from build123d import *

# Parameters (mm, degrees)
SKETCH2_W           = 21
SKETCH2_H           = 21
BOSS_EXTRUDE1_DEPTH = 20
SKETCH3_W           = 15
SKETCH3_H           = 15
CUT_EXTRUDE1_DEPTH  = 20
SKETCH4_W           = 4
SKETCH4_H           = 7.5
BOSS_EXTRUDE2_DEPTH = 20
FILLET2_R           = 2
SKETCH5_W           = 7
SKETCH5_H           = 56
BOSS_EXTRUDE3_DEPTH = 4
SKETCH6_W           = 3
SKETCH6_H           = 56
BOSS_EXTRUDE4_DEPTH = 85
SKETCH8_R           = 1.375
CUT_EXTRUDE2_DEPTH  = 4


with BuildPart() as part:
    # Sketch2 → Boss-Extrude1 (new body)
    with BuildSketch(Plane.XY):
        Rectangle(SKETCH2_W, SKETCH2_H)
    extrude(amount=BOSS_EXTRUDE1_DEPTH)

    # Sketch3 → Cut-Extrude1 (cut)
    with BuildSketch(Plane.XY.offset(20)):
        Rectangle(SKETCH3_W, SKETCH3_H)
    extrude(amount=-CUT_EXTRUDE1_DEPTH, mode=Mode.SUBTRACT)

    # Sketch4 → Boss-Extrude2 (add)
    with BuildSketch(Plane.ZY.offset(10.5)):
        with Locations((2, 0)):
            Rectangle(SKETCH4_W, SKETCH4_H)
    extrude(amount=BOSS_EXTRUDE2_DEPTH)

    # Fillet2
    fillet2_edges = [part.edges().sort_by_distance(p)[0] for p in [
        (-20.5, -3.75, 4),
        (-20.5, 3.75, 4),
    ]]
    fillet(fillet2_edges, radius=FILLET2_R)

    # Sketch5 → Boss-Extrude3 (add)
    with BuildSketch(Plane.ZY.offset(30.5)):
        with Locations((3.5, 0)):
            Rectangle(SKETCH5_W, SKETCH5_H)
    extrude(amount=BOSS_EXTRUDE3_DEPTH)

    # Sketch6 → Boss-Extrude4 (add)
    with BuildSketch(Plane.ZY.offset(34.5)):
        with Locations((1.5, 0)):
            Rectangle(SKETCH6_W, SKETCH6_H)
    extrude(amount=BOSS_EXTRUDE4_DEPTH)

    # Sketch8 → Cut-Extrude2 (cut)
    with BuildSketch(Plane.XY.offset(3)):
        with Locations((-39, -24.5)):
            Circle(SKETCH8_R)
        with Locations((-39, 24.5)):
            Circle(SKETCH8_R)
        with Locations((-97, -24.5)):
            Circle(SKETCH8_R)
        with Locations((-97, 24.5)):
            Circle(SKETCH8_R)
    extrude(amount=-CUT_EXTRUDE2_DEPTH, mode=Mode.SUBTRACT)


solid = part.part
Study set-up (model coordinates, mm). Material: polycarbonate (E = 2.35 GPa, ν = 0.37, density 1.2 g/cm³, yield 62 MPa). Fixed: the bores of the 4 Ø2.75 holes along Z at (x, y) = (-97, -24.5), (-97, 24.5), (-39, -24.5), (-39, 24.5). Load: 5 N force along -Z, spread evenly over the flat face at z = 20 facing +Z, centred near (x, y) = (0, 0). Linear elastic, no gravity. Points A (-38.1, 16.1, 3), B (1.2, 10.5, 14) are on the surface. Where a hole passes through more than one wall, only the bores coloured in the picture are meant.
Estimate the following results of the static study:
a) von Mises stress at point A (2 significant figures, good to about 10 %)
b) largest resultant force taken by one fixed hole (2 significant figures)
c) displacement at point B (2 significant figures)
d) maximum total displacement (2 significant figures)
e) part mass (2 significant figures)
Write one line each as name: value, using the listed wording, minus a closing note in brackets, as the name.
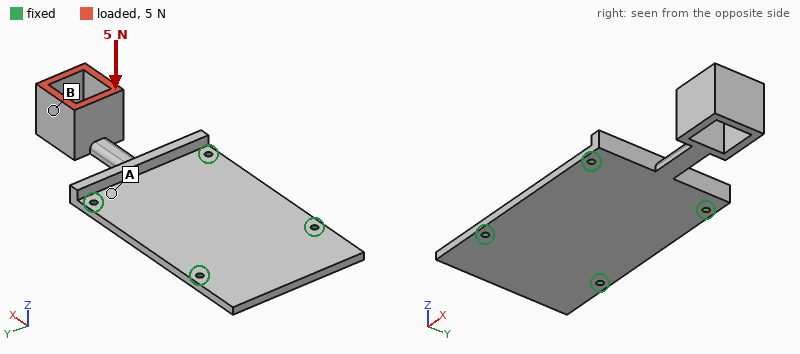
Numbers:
von Mises stress at point A: 1.5 MPa
largest resultant force taken by one fixed hole: 6.8 N
displacement at point B: 1.2 mm
maximum total displacement: 1.6 mm
part mass: 25 g
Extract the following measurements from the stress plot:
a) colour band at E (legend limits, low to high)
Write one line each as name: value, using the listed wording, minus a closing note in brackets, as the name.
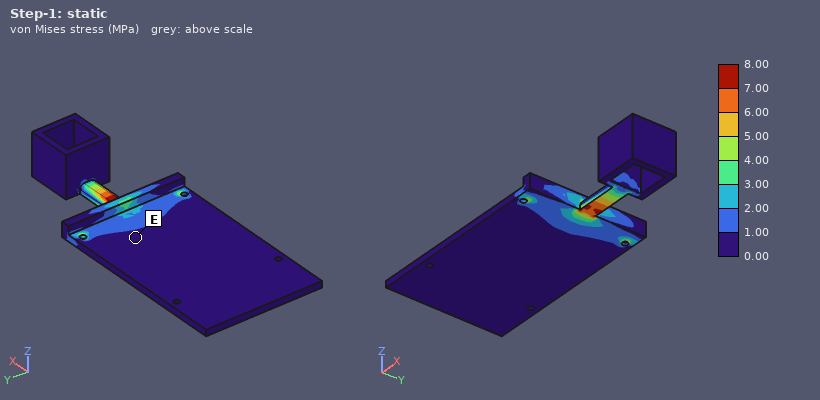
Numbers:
colour band at E: 0.00 to 1.00 MPa
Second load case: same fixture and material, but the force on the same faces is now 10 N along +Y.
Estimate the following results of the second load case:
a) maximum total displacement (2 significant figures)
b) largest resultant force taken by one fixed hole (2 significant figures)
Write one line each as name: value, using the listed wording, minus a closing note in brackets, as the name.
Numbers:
maximum total displacement: 1.6 mm
largest resultant force taken by one fixed hole: 9.3 N
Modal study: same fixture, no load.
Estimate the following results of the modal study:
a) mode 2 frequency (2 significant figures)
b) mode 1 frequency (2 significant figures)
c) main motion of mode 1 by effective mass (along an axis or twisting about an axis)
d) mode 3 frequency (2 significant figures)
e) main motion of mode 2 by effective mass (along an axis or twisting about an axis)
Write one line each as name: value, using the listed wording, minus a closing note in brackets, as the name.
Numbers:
mode 2 frequency: 250 Hz
mode 1 frequency: 140 Hz
main motion of mode 1 by effective mass: along Z
mode 3 frequency: 480 Hz
main motion of mode 2 by effective mass: along Y
